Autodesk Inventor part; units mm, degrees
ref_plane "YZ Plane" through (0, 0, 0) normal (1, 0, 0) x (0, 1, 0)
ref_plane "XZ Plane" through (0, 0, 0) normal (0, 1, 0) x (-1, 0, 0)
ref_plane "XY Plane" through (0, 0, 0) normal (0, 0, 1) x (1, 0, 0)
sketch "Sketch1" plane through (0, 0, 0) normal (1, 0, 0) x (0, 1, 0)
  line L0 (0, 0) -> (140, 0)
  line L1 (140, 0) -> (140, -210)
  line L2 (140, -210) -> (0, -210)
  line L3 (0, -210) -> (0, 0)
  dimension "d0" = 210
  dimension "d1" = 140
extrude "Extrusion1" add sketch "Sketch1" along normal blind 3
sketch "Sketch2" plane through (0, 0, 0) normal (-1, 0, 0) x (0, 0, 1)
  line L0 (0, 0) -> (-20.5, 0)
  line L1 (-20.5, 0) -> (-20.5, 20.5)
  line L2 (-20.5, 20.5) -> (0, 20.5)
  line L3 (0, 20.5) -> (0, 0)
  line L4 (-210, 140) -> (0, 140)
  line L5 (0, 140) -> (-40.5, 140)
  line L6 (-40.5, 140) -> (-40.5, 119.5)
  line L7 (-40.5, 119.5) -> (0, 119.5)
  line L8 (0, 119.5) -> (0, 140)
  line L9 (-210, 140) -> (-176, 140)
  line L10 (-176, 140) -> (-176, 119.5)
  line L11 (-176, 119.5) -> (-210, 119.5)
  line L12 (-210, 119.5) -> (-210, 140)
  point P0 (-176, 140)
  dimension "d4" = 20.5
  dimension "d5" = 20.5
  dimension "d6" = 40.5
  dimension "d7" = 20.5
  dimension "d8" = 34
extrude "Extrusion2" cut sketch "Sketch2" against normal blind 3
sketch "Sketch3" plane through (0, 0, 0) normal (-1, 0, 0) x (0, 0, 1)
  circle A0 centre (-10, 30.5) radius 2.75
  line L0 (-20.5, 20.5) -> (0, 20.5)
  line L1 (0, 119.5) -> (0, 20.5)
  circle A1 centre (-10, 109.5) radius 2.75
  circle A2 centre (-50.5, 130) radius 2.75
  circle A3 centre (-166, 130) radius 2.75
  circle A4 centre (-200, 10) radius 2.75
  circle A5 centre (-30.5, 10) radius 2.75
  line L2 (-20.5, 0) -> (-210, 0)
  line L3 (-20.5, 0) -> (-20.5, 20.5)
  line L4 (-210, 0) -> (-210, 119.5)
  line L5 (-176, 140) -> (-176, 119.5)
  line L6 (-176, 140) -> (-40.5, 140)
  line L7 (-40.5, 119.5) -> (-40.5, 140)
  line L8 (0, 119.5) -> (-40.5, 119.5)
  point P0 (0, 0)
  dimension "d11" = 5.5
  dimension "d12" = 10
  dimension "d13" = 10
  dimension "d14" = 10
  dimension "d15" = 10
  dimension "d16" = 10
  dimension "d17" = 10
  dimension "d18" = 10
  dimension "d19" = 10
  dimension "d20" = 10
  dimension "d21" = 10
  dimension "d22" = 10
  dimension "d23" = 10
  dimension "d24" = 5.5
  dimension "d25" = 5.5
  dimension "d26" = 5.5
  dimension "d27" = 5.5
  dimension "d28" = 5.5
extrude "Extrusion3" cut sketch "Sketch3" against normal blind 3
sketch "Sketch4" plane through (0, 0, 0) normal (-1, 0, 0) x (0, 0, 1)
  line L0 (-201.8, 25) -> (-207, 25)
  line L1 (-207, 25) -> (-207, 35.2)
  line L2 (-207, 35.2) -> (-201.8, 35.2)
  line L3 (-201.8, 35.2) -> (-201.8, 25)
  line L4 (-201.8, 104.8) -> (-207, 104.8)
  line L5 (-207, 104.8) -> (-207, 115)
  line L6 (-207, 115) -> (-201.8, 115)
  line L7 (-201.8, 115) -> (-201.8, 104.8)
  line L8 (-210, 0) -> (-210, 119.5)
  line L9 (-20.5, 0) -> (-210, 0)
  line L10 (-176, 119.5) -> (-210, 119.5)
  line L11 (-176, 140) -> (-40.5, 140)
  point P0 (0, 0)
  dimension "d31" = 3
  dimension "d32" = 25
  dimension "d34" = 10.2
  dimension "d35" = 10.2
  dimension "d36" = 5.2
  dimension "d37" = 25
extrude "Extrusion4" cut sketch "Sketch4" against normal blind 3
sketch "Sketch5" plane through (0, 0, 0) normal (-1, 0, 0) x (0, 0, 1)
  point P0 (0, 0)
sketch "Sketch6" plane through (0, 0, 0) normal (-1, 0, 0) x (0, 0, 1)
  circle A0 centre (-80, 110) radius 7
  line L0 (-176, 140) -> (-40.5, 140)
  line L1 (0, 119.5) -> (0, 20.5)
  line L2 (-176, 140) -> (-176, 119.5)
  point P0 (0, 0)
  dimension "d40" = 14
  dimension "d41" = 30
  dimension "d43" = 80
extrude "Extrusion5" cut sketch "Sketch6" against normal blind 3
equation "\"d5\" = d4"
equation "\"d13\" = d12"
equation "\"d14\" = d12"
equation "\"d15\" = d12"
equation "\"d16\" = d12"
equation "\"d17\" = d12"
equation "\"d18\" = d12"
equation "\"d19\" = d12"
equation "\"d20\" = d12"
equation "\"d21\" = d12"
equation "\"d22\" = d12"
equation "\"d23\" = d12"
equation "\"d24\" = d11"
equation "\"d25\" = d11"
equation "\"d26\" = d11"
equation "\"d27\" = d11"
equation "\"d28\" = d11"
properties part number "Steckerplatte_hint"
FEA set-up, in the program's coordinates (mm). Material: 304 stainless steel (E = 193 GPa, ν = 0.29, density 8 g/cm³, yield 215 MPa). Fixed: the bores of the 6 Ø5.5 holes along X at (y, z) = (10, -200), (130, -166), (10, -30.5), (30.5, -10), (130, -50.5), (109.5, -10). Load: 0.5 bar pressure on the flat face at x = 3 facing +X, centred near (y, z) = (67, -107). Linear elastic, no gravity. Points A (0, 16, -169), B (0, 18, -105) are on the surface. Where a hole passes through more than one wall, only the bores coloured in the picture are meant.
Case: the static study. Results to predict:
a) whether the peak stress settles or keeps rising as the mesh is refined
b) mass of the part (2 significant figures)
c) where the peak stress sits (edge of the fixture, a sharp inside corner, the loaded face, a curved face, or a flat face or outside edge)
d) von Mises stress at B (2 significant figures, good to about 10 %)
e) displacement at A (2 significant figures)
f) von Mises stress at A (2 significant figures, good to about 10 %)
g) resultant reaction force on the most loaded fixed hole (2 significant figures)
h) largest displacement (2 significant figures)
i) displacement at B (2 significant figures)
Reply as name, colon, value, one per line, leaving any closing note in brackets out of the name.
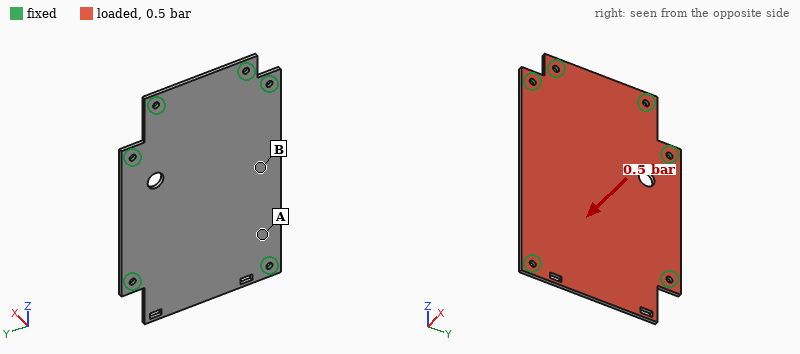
whether the peak stress settles or keeps rising as the mesh is refined: keeps rising
mass of the part: 650 g
where the peak stress sits: edge of the fixture
von Mises stress at B: 39 MPa
displacement at A: 0.13 mm
von Mises stress at A: 17 MPa
resultant reaction force on the most loaded fixed hole: 340 N
largest displacement: 0.31 mm
displacement at B: 0.29 mm
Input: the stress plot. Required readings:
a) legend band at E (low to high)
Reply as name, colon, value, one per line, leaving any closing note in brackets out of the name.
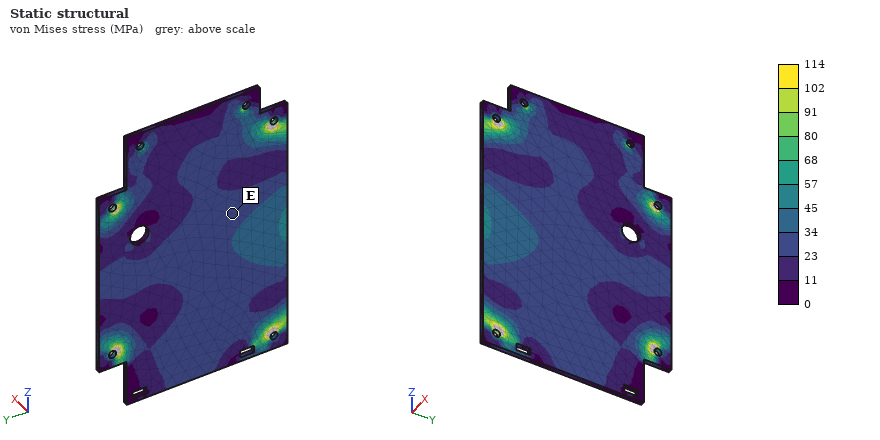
legend band at E: 23 to 34 MPa
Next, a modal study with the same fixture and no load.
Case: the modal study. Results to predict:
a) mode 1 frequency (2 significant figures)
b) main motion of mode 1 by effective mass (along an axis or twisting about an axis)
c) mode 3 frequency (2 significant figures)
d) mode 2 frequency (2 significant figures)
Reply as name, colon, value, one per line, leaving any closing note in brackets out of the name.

mode 1 frequency: 510 Hz
main motion of mode 1 by effective mass: along X
mode 3 frequency: 970 Hz
mode 2 frequency: 830 Hz
